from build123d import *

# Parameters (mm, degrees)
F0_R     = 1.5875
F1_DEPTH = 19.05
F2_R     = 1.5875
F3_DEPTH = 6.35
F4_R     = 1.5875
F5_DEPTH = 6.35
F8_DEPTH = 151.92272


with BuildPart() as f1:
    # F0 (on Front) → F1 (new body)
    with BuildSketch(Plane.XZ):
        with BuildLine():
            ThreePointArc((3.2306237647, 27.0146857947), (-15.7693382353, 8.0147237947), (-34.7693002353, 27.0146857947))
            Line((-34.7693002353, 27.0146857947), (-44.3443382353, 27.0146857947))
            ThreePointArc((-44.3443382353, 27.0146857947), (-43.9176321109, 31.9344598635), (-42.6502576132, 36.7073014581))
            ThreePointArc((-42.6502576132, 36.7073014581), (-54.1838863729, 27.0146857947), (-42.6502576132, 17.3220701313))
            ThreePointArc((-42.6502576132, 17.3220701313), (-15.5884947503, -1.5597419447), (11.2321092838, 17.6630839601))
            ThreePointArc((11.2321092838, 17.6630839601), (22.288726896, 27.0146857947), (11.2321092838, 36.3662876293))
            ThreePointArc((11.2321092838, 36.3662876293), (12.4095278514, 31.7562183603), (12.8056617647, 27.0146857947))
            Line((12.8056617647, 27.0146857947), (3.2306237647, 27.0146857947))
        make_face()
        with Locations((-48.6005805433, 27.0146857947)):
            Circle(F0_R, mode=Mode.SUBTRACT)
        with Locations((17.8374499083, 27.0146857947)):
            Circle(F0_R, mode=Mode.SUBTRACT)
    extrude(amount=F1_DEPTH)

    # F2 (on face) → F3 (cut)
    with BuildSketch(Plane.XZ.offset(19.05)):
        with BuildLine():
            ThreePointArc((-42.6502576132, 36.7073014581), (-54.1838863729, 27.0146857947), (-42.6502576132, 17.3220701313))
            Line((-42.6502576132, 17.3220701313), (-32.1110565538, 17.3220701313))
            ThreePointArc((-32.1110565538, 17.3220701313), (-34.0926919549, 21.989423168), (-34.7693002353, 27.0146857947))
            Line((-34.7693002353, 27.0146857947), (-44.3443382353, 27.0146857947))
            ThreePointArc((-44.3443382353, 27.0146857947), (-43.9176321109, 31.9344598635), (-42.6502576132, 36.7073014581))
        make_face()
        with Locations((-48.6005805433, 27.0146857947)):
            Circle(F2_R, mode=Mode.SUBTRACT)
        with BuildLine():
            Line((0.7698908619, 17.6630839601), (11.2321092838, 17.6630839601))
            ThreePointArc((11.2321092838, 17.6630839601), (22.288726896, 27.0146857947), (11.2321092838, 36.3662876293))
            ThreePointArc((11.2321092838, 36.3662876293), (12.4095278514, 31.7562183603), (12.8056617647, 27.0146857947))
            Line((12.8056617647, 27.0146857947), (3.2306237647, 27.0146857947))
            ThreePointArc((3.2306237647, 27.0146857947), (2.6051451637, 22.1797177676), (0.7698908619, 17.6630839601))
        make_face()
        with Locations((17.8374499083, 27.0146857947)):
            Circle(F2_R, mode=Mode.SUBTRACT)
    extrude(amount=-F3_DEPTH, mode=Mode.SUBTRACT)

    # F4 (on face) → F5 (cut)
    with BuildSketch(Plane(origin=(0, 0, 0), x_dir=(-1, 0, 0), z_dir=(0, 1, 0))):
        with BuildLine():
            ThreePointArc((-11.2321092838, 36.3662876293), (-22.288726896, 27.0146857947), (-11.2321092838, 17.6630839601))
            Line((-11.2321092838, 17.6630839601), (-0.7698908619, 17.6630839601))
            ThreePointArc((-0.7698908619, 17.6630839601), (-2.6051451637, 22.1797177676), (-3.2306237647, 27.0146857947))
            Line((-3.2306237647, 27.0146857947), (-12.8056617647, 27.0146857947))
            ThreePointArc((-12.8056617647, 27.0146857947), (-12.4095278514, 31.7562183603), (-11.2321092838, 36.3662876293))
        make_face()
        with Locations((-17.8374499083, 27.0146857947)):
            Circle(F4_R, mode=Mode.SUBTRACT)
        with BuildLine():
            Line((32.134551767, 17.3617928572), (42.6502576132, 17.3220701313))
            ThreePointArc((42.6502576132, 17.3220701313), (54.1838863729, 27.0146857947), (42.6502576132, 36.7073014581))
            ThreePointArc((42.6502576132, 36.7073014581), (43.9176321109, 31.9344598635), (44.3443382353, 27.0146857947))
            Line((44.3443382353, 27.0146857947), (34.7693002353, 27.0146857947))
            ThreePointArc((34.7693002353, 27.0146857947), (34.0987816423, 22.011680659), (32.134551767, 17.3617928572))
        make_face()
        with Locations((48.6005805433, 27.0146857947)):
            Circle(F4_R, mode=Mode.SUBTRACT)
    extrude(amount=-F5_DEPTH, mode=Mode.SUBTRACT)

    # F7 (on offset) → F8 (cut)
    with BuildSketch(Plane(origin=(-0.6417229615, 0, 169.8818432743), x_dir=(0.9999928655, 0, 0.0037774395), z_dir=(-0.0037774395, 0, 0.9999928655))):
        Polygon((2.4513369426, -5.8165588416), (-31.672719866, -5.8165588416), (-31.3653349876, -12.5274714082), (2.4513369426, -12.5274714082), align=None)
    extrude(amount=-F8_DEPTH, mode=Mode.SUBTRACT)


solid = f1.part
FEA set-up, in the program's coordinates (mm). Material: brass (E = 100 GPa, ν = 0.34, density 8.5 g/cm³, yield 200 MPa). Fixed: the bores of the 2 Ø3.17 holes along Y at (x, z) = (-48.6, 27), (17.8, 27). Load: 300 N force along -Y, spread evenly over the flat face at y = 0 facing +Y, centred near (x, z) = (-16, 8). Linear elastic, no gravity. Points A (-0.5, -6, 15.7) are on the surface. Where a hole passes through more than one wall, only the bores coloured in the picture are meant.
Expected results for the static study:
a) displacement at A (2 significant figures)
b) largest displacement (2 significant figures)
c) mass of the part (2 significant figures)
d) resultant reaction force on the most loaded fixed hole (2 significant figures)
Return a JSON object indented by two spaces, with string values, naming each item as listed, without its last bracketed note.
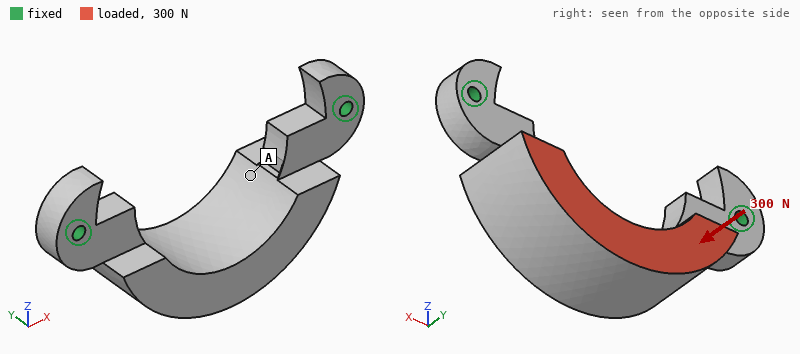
{
  "displacement at A": "16 µm",
  "largest displacement": "49 µm",
  "mass of the part": "110 g",
  "resultant reaction force on the most loaded fixed hole": "150 N"
}
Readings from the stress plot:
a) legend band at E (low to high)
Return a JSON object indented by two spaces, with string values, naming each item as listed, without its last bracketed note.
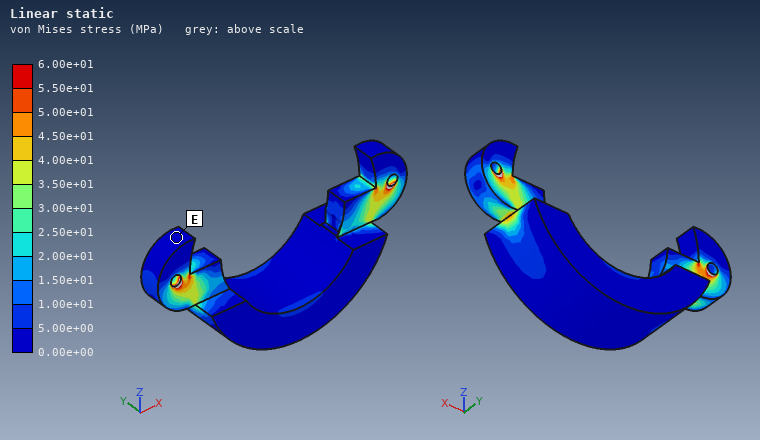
{
  "legend band at E": "0.00e+00 to 5.00e+00 MPa"
}
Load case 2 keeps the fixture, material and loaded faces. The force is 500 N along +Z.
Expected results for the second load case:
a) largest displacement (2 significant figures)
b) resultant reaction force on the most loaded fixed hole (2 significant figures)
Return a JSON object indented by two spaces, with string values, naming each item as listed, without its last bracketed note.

{
  "largest displacement": "53 µm",
  "resultant reaction force on the most loaded fixed hole": "320 N"
}
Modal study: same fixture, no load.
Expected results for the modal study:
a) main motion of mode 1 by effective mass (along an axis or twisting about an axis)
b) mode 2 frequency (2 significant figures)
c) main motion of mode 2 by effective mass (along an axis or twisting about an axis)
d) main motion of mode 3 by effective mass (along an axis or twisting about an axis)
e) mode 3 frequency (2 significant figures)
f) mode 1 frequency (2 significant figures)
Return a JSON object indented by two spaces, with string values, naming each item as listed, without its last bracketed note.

{
  "main motion of mode 1 by effective mass": "along Y",
  "mode 2 frequency": "6600 Hz",
  "main motion of mode 2 by effective mass": "along X",
  "main motion of mode 3 by effective mass": "twisting about Z",
  "mode 3 frequency": "7900 Hz",
  "mode 1 frequency": "1600 Hz"
}
